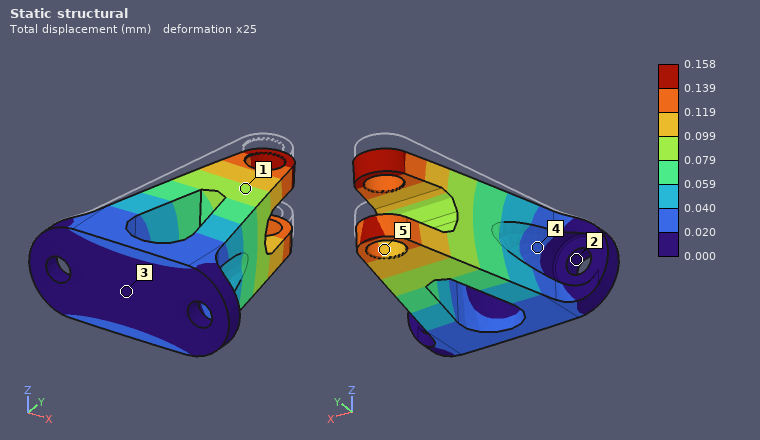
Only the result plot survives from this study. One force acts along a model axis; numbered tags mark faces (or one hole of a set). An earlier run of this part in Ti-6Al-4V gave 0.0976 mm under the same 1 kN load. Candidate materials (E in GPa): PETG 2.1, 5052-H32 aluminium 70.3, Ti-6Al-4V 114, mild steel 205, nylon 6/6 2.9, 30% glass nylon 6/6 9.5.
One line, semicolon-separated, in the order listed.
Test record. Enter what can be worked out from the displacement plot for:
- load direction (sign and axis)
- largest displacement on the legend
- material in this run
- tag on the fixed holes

-Z; 0.158 mm; 5052-H32 aluminium; 2
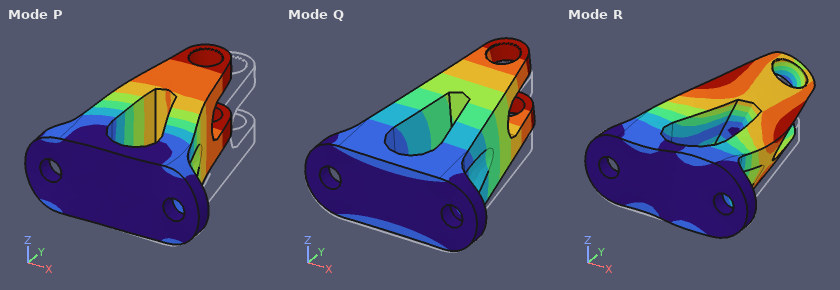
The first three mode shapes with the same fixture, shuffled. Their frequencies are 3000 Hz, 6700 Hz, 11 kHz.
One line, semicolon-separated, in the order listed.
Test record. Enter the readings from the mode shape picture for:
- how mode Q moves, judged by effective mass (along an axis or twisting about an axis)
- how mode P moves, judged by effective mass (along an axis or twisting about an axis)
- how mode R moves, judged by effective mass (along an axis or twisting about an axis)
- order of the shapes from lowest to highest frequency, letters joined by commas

along Z; along X; twisting about Y; Q, P, R
